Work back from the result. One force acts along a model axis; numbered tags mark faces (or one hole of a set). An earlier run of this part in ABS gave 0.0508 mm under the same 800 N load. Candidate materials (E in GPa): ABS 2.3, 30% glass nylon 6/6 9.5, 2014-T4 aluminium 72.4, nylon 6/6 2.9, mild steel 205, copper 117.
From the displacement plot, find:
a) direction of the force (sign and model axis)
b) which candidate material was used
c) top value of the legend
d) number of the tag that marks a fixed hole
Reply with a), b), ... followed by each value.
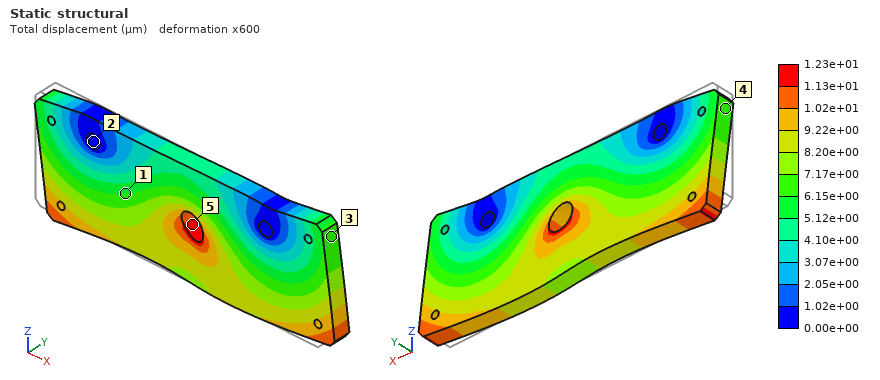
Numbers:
a) +X
b) 30% glass nylon 6/6
c) 1.23e+01 µm
d) 2
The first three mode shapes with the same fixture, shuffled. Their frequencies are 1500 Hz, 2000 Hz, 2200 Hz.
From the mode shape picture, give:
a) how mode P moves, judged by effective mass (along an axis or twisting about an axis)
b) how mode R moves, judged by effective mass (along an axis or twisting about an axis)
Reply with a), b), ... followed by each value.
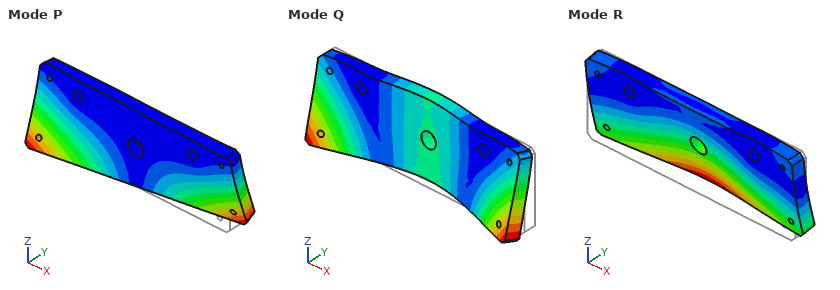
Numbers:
a) twisting about Z
b) along Y
